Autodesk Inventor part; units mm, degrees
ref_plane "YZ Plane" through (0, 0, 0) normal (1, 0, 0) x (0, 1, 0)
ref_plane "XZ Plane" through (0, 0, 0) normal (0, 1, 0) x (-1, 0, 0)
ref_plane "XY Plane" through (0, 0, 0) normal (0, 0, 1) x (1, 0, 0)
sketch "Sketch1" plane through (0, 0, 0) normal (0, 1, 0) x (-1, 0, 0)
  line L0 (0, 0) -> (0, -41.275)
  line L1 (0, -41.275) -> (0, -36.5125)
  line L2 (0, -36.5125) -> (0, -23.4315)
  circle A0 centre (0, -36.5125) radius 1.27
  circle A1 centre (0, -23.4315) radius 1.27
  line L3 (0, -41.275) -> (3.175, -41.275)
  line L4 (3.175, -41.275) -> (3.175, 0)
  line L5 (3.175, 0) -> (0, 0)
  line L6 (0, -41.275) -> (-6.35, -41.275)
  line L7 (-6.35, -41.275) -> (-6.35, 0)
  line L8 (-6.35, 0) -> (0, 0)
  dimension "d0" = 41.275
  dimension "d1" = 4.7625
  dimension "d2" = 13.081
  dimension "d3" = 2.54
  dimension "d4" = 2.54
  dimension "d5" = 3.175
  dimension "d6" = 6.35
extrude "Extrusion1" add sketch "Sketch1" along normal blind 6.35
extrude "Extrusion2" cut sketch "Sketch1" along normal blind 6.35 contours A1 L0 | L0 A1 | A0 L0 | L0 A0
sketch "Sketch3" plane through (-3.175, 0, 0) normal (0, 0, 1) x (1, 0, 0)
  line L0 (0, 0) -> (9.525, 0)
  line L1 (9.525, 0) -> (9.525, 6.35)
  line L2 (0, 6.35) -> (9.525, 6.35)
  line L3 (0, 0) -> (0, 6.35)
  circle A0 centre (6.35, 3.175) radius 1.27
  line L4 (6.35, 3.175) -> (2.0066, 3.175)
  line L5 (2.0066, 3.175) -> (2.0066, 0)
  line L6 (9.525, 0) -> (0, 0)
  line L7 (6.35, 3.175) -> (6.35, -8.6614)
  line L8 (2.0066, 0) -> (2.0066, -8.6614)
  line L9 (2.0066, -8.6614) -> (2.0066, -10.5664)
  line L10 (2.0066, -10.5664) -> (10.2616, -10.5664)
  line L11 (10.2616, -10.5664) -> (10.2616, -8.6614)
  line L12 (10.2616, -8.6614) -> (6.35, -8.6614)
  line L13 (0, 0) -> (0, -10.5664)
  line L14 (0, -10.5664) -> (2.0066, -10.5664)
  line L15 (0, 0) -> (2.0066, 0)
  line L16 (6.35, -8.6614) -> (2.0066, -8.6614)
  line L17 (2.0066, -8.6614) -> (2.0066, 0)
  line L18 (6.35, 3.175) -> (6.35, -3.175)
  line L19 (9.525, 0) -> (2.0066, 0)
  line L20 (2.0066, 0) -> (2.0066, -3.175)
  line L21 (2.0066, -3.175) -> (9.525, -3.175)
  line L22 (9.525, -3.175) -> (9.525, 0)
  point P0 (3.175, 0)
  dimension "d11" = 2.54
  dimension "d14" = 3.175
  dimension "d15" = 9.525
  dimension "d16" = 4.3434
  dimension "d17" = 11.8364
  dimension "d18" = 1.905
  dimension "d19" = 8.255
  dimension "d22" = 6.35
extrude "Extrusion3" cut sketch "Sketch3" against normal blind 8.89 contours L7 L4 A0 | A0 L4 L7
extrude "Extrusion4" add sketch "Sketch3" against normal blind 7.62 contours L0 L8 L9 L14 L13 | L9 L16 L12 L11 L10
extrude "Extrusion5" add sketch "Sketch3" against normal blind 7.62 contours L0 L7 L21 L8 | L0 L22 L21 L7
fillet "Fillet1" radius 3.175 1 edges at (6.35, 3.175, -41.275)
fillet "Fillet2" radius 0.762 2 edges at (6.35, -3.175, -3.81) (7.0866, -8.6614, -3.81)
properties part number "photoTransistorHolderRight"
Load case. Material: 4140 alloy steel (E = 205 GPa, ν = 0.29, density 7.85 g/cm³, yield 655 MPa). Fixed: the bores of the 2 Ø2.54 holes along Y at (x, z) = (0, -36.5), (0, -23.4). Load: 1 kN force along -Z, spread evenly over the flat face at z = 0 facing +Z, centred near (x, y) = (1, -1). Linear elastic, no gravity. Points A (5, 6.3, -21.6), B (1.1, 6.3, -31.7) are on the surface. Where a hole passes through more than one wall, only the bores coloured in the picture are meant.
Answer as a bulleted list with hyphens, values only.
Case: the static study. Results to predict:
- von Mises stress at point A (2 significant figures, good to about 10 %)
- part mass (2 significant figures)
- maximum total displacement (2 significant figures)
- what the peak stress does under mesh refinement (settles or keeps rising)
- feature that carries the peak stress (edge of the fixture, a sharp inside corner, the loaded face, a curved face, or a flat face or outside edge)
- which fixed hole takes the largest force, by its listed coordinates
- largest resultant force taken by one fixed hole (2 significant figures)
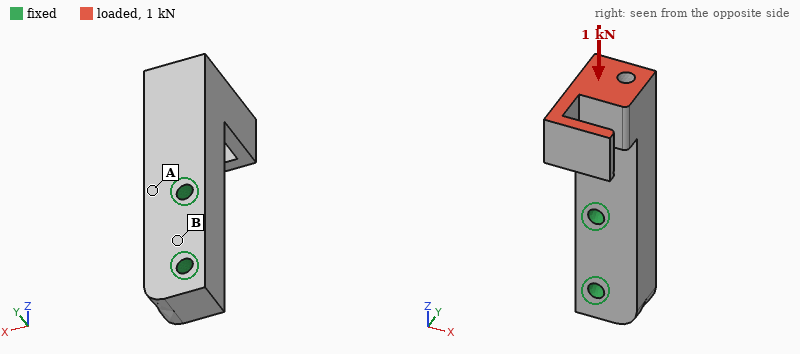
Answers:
- 35 MPa
- 22 g
- 67 µm
- keeps rising
- edge of the fixture
- (0, -23.4)
- 880 N
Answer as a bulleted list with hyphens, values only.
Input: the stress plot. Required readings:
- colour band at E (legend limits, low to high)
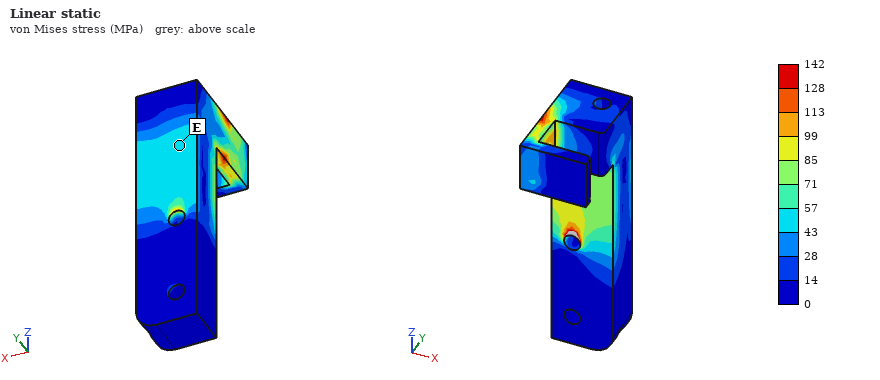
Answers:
- 43 to 57 MPa
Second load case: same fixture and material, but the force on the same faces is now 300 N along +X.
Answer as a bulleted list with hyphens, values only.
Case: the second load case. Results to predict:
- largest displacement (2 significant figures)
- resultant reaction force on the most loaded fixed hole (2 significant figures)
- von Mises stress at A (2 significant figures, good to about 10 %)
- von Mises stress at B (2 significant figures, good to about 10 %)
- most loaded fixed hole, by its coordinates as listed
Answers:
- 48 µm
- 710 N
- 48 MPa
- 17 MPa
- (0, -23.4)
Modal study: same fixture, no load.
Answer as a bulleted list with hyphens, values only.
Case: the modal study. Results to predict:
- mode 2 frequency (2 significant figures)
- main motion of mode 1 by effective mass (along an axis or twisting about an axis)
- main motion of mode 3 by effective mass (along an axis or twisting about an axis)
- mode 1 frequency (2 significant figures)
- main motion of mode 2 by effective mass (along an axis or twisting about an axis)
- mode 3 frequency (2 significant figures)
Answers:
- 6800 Hz
- along Y
- along X
- 5900 Hz
- along X
- 9700 Hz
